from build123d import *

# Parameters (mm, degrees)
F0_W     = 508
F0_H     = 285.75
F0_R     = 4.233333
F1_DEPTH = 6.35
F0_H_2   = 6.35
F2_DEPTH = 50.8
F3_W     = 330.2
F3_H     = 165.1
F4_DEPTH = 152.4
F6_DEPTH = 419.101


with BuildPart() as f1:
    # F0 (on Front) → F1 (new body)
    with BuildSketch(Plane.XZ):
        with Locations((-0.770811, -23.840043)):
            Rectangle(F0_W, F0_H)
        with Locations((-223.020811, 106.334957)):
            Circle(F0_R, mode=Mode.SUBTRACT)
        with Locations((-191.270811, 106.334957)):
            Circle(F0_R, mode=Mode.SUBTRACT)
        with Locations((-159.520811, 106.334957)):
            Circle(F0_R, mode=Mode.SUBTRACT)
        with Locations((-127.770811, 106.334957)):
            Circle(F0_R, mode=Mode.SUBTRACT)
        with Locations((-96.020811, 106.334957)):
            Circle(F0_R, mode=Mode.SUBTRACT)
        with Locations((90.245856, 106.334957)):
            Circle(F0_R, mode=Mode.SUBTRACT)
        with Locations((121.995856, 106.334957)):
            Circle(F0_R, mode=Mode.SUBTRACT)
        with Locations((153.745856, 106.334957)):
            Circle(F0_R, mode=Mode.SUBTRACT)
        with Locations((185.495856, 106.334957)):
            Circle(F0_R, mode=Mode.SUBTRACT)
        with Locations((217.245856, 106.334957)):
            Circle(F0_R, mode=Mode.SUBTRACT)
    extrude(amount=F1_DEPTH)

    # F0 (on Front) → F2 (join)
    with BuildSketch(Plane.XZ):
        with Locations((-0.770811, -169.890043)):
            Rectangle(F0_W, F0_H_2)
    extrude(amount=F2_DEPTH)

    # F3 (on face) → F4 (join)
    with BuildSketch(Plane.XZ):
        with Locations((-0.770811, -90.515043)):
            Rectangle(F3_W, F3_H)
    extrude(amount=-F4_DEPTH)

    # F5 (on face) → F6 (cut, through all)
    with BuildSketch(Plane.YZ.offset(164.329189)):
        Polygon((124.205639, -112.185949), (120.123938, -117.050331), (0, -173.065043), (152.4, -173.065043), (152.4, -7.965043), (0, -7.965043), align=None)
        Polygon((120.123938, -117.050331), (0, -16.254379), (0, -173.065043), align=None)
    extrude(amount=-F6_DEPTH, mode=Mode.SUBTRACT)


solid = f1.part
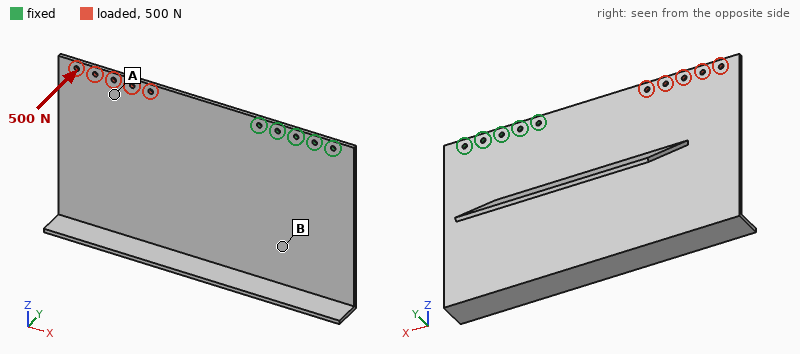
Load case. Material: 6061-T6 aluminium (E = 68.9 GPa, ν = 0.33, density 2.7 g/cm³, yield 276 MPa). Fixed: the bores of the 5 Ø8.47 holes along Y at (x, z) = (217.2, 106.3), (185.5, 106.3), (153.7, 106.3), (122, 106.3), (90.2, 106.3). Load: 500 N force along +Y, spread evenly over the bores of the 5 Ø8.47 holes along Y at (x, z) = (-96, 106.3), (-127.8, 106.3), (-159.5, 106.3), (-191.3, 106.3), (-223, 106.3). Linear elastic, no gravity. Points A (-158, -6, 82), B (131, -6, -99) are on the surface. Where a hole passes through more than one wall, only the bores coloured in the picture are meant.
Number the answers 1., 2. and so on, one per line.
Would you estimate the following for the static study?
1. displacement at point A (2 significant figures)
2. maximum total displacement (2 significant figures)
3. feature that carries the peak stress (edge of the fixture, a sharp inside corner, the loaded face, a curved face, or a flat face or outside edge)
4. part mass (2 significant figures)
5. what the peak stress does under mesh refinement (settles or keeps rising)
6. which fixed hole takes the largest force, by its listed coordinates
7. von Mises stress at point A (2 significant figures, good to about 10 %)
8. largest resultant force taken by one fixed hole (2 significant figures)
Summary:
1. 4.7 mm
2. 7.0 mm
3. edge of the fixture
4. 3.8 kg
5. keeps rising
6. (90.2, 106.3)
7. 20 MPa
8. 1.6 kN
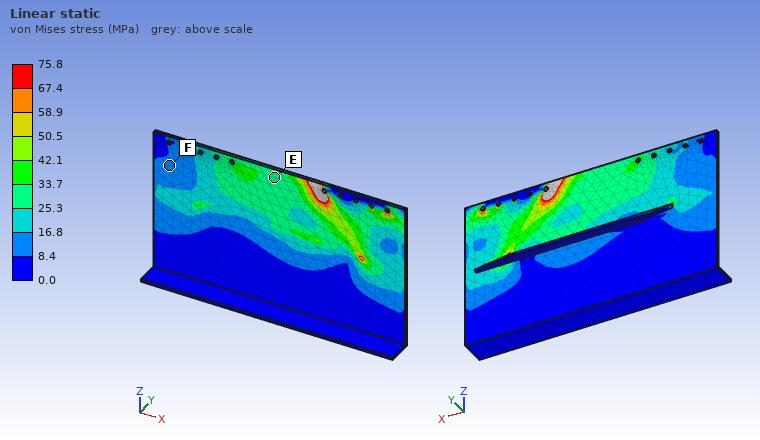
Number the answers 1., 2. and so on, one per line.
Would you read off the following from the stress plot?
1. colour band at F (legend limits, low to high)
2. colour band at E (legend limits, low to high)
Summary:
1. 8.4 to 16.8 MPa
2. 25.3 to 33.7 MPa
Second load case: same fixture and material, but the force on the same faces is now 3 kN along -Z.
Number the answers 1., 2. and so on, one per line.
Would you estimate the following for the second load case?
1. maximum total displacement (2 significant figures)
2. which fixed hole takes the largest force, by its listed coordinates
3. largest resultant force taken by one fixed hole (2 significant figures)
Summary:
1. 0.28 mm
2. (90.2, 106.3)
3. 7.7 kN
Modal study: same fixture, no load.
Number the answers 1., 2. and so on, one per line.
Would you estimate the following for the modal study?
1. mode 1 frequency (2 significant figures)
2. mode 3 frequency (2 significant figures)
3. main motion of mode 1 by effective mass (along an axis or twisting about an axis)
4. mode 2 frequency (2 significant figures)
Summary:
1. 26 Hz
2. 120 Hz
3. along Y
4. 60 Hz
